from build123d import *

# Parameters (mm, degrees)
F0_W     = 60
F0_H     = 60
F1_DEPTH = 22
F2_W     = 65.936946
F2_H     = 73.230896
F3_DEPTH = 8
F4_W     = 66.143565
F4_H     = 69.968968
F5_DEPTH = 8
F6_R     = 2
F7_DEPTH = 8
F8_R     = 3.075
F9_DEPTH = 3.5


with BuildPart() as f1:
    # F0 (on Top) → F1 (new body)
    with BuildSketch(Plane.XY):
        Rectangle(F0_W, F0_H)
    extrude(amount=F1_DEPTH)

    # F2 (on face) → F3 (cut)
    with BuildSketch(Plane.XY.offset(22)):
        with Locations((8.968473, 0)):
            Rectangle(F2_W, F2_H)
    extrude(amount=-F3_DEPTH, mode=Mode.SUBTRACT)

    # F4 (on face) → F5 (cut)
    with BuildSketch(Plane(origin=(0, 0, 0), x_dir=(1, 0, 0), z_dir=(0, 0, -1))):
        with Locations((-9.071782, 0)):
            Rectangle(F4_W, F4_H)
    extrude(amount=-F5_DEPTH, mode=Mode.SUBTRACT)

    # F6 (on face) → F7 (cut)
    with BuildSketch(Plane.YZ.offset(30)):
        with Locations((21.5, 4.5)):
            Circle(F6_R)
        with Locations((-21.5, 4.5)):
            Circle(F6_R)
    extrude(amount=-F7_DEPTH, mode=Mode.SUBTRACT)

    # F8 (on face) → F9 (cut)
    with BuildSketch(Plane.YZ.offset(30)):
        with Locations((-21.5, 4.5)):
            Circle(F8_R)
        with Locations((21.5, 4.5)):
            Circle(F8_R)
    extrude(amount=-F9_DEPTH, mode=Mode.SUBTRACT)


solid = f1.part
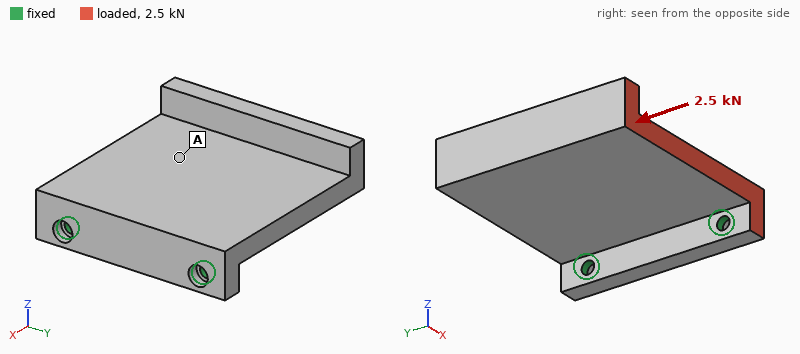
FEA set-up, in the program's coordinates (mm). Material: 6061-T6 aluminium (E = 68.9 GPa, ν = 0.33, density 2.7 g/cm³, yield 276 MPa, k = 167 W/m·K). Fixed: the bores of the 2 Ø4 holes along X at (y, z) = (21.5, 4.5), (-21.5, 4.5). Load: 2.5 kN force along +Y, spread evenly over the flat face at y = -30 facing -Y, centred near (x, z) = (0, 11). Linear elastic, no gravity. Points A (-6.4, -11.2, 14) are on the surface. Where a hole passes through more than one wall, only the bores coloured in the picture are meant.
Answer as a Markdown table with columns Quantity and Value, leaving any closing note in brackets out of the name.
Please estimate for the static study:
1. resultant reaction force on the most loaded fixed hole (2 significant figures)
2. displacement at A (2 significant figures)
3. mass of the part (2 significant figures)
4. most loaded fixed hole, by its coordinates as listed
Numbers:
| Quantity | Value |
|---|---|
| resultant reaction force on the most loaded fixed hole | 2.0 kN |
| displacement at A | 38 µm |
| mass of the part | 73 g |
| most loaded fixed hole, by its coordinates as listed | (-21.5, 4.5) |
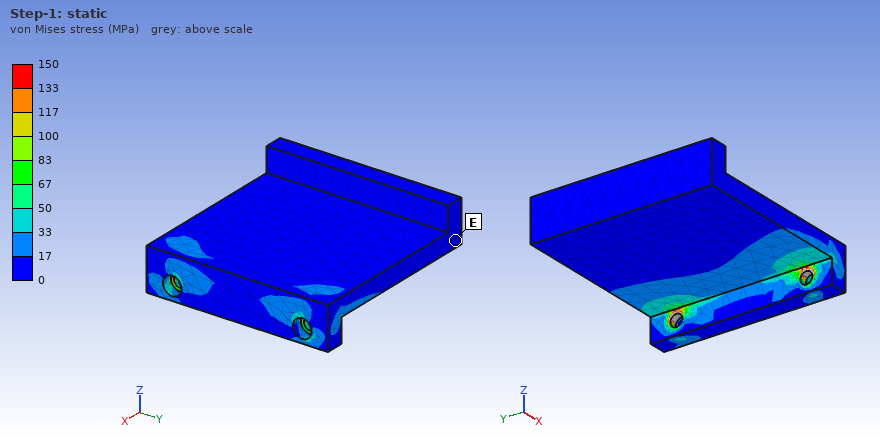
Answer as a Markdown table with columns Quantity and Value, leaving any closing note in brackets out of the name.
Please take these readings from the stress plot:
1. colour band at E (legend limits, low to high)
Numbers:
| Quantity | Value |
|---|---|
| colour band at E | 0 to 17 MPa |
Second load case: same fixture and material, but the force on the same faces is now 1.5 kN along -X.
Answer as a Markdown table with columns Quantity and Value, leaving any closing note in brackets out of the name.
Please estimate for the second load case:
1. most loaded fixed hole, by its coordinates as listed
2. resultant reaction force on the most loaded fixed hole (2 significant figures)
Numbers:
| Quantity | Value |
|---|---|
| most loaded fixed hole, by its coordinates as listed | (-21.5, 4.5) |
| resultant reaction force on the most loaded fixed hole | 1.8 kN |
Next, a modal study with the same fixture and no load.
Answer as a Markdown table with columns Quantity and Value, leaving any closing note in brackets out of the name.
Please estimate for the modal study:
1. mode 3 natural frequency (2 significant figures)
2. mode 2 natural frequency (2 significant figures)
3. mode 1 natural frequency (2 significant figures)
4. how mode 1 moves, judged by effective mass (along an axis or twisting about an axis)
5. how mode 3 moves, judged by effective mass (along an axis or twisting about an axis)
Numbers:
| Quantity | Value |
|---|---|
| mode 3 natural frequency | 4200 Hz |
| mode 2 natural frequency | 2700 Hz |
| mode 1 natural frequency | 740 Hz |
| how mode 1 moves, judged by effective mass | along Z |
| how mode 3 moves, judged by effective mass | along Y |
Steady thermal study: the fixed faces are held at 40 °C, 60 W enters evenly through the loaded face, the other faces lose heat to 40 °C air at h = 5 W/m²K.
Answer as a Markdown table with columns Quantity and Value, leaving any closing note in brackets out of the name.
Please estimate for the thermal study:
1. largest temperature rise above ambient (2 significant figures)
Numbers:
| Quantity | Value |
|---|---|
| largest temperature rise above ambient | 56 K |
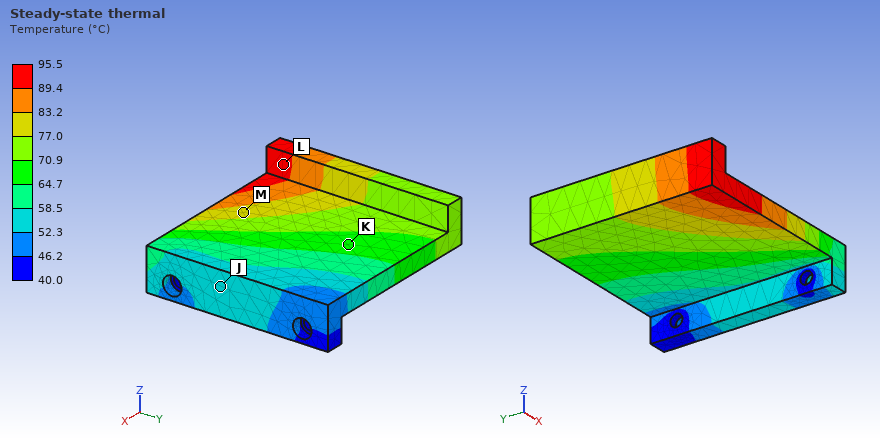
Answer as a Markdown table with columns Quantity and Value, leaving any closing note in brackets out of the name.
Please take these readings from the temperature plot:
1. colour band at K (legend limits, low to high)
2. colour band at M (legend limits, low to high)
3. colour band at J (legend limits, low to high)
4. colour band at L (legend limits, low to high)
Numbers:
| Quantity | Value |
|---|---|
| colour band at K | 64.7 to 70.9 °C |
| colour band at M | 77.0 to 83.2 °C |
| colour band at J | 52.3 to 58.5 °C |
| colour band at L | 89.4 to 95.5 °C |
